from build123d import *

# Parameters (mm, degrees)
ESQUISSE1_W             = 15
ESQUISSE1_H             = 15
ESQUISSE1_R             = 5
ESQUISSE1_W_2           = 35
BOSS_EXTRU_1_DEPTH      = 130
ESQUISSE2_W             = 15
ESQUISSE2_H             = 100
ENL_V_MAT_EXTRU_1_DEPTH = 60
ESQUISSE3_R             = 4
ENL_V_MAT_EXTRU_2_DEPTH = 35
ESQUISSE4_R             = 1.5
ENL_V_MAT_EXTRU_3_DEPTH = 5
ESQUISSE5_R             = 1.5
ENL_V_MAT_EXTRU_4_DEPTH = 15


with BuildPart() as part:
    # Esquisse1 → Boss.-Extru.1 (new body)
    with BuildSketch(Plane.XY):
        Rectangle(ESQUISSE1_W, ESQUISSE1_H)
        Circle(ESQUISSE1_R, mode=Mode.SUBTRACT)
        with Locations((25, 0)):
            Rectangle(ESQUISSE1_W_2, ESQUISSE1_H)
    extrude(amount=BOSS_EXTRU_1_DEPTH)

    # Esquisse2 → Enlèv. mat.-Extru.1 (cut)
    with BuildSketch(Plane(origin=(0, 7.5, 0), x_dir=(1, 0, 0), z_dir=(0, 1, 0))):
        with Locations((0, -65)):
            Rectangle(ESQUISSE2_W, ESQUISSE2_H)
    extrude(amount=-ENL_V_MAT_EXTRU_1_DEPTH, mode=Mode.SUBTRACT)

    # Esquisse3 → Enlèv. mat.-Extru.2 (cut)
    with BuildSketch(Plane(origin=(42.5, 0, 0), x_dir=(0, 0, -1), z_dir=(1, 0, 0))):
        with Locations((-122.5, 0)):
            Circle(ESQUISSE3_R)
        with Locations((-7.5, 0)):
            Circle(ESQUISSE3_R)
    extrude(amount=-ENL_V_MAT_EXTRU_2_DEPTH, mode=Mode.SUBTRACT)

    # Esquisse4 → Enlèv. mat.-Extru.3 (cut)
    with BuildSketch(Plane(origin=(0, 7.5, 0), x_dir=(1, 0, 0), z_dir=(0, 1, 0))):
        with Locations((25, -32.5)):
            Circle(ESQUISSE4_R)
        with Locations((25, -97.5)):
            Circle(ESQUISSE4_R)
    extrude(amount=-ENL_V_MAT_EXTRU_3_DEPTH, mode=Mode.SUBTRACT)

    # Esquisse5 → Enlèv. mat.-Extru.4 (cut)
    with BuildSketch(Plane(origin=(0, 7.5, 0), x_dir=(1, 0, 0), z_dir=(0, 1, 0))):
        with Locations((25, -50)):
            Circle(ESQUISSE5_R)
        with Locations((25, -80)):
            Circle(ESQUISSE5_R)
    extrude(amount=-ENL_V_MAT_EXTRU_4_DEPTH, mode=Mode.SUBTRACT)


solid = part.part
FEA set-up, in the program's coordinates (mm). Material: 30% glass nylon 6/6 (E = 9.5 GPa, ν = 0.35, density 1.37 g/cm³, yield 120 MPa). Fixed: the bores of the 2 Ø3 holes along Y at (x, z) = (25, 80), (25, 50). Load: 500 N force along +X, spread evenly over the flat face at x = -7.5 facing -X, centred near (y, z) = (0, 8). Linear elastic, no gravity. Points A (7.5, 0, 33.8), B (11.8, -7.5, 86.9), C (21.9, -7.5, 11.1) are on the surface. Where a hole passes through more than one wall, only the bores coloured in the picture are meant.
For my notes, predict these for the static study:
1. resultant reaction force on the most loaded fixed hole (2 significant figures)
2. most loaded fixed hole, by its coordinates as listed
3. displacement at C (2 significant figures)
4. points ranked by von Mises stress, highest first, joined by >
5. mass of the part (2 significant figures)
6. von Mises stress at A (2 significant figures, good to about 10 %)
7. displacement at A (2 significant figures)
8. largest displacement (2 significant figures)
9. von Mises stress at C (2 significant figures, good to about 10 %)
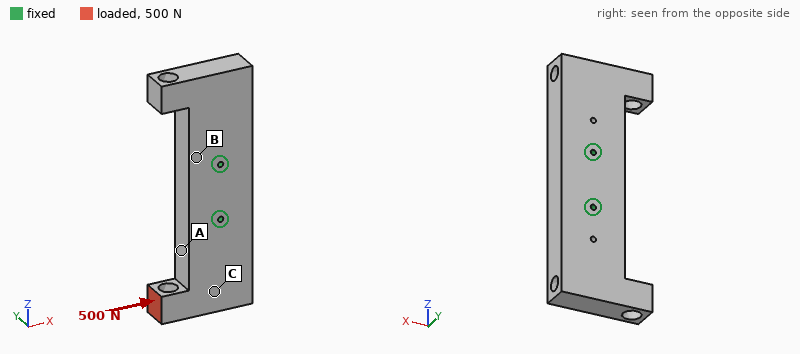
1.2 kN
(25, 50)
0.073 mm
A > C > B
94 g
4.7 MPa
0.039 mm
0.14 mm
2.7 MPa
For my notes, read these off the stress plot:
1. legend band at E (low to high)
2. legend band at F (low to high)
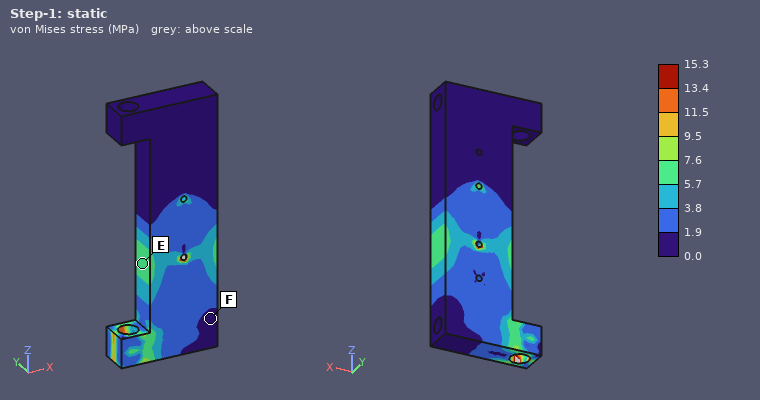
5.7 to 7.6 MPa
0.0 to 1.9 MPa
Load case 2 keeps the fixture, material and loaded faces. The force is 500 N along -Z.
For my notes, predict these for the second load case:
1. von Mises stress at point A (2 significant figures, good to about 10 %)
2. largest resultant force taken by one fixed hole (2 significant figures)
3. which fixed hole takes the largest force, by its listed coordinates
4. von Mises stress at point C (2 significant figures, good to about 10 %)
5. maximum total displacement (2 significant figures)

6.1 MPa
620 N
(25, 50)
4.5 MPa
0.21 mm
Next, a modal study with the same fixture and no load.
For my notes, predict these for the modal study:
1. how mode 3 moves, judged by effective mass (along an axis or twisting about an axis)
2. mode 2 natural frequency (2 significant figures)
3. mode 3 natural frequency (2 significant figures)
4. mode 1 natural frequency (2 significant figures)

twisting about Y
2000 Hz
2600 Hz
1900 Hz
